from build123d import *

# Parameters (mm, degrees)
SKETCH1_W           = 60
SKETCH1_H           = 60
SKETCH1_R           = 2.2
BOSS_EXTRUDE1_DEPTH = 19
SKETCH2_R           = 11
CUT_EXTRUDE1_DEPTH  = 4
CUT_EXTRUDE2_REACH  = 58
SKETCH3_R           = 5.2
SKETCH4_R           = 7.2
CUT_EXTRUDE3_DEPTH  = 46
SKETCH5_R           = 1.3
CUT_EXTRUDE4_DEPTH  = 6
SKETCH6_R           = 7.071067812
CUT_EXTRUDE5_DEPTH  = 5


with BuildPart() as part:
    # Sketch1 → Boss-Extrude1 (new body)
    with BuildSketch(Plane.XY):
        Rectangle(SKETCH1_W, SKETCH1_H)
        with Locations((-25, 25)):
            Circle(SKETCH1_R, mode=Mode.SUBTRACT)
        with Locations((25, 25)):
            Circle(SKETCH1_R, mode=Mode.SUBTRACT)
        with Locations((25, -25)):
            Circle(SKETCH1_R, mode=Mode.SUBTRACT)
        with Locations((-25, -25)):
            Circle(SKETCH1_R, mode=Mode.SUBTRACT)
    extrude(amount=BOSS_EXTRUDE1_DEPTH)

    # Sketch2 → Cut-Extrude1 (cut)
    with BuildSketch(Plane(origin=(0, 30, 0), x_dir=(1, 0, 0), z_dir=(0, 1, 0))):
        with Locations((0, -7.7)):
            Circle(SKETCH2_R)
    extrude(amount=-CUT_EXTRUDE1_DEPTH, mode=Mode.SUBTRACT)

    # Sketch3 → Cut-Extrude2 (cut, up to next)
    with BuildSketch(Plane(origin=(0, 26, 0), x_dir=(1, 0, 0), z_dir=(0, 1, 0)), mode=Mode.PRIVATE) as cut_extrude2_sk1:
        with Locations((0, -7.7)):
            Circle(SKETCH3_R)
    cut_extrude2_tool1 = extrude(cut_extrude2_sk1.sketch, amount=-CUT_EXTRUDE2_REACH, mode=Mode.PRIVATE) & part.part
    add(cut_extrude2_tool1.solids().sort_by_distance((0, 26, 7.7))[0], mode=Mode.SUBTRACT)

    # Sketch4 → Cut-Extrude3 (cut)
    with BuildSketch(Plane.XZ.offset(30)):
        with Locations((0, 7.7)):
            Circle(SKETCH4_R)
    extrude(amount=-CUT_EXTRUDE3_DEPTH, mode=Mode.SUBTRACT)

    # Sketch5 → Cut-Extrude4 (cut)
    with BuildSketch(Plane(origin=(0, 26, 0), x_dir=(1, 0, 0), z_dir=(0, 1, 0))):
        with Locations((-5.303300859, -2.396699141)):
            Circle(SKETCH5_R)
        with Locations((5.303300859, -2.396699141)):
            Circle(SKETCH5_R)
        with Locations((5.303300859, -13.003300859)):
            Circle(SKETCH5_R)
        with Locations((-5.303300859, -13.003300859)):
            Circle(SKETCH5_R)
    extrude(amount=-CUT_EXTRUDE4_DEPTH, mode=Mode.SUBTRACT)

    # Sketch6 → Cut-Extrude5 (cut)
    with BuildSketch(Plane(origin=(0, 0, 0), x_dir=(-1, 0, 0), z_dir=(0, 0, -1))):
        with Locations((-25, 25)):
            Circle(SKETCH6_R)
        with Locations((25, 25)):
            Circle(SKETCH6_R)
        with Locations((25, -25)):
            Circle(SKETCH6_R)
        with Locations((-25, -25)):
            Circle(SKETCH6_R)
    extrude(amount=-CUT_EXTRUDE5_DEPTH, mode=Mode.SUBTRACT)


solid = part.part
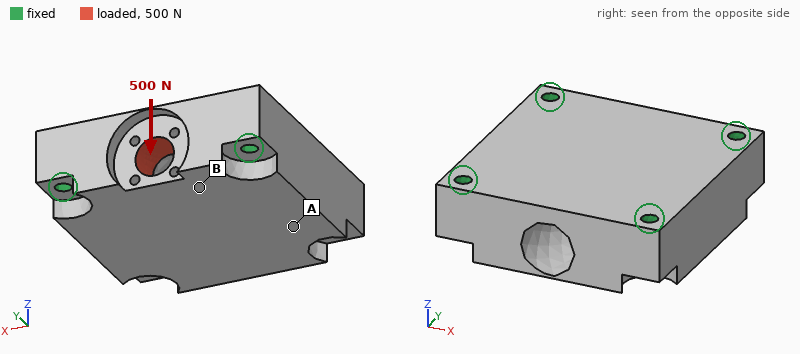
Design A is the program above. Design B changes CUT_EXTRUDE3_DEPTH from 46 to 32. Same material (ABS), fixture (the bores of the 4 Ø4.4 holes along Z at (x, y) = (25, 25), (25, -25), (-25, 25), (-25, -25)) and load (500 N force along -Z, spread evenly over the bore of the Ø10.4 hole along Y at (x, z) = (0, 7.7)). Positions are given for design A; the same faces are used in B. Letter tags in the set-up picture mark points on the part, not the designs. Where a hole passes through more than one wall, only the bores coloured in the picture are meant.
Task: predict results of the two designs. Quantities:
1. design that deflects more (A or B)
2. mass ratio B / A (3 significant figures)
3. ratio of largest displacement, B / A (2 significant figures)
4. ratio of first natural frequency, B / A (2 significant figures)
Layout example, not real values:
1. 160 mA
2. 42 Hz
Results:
1. A
2. 1.02
3. 0.58
4. 1.00
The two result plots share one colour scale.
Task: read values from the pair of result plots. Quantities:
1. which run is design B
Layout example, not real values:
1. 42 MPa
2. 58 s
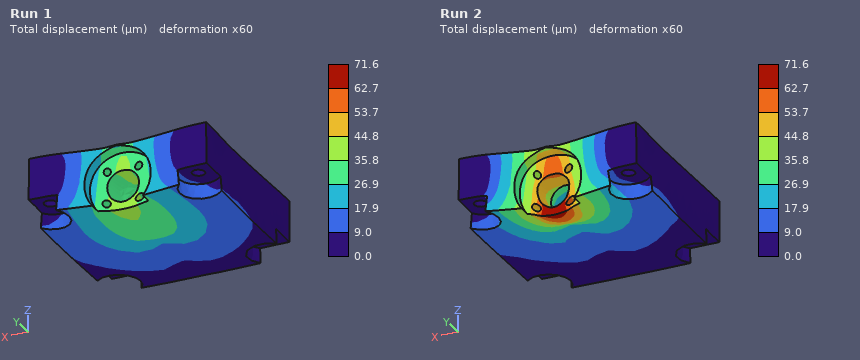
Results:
1. Run 1
